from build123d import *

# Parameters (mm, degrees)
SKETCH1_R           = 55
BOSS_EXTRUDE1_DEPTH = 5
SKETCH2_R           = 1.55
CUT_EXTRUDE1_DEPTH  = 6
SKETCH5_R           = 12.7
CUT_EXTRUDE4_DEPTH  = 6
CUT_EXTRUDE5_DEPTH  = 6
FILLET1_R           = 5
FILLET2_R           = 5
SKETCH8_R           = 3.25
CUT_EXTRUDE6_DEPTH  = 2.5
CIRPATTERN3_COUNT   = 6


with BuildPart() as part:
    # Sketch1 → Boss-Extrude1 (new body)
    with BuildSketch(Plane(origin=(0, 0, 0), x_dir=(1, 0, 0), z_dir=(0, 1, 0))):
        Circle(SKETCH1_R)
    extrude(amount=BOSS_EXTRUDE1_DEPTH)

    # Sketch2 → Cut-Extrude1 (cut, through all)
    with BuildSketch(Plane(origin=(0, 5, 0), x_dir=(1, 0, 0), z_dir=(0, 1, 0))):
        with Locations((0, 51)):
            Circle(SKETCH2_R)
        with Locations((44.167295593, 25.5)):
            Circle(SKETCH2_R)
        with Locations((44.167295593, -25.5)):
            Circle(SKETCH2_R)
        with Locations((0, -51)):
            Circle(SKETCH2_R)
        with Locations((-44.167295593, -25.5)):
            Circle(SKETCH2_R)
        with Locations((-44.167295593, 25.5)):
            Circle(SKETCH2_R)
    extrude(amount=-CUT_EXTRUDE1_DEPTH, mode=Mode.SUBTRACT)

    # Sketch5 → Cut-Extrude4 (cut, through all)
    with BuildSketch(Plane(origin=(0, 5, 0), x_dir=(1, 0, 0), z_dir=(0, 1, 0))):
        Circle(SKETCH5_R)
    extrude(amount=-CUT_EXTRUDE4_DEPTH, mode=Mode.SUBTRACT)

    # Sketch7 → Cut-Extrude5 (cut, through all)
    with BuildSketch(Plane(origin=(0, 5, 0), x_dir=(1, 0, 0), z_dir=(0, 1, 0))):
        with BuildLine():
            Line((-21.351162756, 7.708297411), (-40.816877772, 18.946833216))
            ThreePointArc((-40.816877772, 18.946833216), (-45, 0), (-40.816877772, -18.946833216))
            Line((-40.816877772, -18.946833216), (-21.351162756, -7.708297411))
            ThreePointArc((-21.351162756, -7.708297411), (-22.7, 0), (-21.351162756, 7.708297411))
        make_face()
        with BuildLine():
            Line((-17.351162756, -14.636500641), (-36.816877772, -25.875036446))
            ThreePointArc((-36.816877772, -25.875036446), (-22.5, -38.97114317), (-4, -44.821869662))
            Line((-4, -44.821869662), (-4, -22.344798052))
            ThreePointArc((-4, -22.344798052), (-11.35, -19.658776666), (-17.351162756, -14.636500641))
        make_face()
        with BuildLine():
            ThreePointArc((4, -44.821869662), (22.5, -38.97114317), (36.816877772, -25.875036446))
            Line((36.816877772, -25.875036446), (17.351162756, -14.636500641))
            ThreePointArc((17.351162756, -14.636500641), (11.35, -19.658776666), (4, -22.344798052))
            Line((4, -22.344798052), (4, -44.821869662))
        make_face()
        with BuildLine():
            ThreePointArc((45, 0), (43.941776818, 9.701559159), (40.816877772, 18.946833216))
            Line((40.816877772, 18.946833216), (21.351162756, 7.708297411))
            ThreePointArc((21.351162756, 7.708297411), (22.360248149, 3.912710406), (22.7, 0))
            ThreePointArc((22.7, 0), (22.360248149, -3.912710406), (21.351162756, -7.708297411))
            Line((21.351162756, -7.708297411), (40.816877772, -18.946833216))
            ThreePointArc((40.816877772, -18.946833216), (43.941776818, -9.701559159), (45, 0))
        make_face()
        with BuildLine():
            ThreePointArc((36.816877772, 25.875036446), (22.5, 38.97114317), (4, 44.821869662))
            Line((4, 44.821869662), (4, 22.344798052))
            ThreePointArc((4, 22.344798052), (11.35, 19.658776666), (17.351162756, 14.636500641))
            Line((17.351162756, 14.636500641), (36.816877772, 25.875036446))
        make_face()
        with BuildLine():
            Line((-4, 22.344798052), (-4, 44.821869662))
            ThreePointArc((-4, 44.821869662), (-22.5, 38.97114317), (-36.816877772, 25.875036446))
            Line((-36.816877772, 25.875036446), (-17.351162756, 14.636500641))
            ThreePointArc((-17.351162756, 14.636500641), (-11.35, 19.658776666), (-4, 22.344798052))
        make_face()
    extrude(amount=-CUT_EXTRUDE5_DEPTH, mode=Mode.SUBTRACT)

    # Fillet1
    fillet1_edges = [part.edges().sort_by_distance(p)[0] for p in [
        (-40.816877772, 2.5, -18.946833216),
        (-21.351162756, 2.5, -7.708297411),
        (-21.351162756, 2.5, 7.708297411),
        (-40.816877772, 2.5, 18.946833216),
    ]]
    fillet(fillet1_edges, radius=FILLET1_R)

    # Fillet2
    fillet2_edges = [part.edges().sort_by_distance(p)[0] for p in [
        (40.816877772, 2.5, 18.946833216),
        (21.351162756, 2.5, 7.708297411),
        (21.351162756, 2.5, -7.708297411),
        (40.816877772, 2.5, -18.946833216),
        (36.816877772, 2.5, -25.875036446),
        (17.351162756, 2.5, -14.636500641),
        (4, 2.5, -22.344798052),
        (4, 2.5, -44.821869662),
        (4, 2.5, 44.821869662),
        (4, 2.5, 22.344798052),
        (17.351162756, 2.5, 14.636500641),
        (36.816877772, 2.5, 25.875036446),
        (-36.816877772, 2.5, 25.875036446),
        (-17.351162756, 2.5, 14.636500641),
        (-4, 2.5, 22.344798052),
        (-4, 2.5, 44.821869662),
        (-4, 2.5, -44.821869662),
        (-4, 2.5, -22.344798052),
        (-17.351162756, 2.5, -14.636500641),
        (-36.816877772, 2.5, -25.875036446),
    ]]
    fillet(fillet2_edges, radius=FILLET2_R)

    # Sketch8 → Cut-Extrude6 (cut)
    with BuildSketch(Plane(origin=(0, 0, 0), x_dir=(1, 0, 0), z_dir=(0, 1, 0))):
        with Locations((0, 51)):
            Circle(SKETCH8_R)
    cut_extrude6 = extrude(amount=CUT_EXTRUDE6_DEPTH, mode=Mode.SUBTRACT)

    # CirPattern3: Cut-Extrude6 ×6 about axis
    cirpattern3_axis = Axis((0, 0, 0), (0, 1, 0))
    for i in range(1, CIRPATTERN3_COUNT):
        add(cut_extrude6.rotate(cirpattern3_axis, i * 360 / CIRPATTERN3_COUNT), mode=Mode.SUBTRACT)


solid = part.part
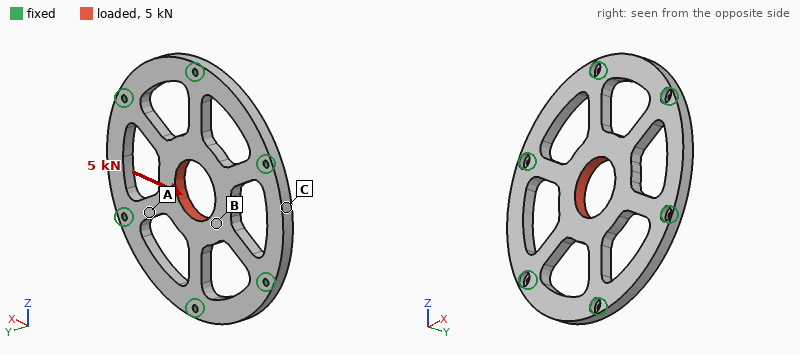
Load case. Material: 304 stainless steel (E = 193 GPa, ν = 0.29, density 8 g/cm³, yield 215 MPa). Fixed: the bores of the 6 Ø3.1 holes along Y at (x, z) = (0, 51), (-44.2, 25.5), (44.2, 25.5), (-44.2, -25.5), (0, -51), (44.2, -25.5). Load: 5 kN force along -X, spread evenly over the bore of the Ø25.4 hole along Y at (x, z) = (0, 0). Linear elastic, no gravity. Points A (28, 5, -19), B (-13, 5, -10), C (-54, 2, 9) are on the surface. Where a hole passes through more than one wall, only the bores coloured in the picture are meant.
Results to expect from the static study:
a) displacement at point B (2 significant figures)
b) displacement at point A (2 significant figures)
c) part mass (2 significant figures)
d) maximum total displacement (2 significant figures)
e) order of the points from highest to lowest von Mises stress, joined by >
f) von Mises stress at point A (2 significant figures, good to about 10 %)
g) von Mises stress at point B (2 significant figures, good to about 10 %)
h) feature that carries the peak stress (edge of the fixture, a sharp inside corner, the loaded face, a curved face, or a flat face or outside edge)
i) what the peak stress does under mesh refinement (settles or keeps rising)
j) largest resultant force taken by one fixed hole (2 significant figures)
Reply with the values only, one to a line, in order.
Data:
7.6 µm
4.9 µm
210 g
8.8 µm
A > B > C
43 MPa
21 MPa
edge of the fixture
keeps rising
1.2 kN
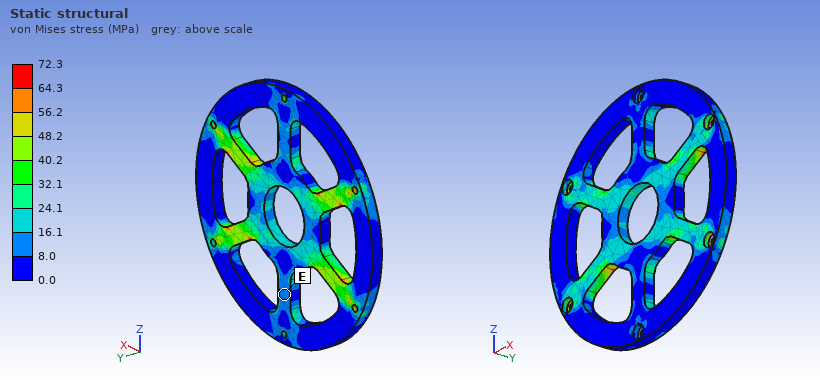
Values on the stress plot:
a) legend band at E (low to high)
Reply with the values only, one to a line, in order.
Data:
8.0 to 16.1 MPa
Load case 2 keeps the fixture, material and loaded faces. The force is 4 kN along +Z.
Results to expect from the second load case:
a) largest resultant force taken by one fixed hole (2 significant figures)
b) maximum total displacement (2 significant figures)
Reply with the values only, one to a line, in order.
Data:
1.1 kN
6.8 µm
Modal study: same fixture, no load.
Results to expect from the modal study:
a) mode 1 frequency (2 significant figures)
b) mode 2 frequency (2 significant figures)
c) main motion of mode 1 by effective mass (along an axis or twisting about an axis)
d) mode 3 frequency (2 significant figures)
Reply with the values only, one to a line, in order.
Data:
2700 Hz
5700 Hz
along Y
5700 Hz
